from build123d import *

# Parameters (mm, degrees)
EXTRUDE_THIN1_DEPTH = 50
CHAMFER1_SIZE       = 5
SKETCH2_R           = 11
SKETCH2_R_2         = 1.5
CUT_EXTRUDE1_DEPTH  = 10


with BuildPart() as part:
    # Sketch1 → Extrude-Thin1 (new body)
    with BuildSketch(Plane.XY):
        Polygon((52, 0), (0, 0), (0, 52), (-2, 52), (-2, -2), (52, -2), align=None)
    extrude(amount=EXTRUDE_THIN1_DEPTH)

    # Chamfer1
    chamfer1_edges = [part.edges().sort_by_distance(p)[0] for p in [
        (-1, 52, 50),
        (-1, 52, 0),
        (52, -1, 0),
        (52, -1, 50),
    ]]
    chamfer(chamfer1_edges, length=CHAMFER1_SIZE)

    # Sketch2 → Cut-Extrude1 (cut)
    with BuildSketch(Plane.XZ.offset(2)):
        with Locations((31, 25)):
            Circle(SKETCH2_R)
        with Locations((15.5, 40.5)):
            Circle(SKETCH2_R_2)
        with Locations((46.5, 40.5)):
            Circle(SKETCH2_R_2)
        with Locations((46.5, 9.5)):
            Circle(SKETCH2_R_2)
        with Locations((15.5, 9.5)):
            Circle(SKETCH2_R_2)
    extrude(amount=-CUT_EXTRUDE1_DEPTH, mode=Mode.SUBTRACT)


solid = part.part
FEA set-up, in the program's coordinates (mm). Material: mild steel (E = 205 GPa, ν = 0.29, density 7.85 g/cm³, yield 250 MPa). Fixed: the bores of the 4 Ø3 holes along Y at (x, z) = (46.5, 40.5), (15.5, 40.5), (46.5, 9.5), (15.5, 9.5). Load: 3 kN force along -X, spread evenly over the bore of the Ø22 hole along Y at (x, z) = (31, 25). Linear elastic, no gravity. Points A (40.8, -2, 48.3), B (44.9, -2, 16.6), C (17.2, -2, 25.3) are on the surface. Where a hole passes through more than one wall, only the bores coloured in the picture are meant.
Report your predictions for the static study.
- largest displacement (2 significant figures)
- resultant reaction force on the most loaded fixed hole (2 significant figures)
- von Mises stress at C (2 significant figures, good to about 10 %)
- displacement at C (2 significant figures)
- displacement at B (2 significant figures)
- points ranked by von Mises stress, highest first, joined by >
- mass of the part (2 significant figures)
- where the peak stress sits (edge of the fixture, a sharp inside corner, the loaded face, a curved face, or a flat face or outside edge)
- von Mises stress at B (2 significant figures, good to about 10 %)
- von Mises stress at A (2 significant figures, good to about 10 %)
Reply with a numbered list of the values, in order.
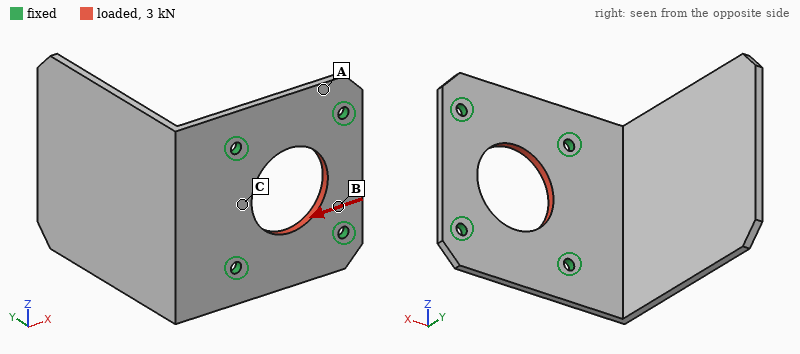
1. 4.8 µm
2. 770 N
3. 19 MPa
4. 2.3 µm
5. 2.6 µm
6. B > C > A
7. 76 g
8. edge of the fixture
9. 31 MPa
10. 7.6 MPa
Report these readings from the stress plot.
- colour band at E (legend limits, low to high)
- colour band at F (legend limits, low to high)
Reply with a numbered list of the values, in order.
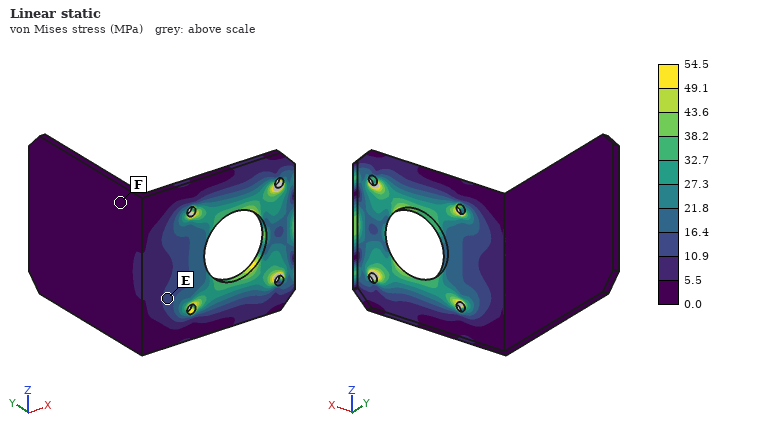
1. 10.9 to 16.4 MPa
2. 0.0 to 5.5 MPa
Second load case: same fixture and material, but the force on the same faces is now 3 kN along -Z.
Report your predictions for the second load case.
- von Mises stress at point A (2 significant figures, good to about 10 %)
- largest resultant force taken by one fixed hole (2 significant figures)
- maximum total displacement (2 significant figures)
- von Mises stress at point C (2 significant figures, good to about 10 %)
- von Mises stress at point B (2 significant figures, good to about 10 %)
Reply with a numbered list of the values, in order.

1. 12 MPa
2. 780 N
3. 3.5 µm
4. 28 MPa
5. 28 MPa
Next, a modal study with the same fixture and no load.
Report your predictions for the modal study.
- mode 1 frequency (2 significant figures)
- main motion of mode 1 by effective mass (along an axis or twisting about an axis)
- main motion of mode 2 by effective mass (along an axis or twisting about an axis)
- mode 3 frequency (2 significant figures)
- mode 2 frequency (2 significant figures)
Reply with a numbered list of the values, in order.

1. 400 Hz
2. along X
3. along Z
4. 1600 Hz
5. 1000 Hz
